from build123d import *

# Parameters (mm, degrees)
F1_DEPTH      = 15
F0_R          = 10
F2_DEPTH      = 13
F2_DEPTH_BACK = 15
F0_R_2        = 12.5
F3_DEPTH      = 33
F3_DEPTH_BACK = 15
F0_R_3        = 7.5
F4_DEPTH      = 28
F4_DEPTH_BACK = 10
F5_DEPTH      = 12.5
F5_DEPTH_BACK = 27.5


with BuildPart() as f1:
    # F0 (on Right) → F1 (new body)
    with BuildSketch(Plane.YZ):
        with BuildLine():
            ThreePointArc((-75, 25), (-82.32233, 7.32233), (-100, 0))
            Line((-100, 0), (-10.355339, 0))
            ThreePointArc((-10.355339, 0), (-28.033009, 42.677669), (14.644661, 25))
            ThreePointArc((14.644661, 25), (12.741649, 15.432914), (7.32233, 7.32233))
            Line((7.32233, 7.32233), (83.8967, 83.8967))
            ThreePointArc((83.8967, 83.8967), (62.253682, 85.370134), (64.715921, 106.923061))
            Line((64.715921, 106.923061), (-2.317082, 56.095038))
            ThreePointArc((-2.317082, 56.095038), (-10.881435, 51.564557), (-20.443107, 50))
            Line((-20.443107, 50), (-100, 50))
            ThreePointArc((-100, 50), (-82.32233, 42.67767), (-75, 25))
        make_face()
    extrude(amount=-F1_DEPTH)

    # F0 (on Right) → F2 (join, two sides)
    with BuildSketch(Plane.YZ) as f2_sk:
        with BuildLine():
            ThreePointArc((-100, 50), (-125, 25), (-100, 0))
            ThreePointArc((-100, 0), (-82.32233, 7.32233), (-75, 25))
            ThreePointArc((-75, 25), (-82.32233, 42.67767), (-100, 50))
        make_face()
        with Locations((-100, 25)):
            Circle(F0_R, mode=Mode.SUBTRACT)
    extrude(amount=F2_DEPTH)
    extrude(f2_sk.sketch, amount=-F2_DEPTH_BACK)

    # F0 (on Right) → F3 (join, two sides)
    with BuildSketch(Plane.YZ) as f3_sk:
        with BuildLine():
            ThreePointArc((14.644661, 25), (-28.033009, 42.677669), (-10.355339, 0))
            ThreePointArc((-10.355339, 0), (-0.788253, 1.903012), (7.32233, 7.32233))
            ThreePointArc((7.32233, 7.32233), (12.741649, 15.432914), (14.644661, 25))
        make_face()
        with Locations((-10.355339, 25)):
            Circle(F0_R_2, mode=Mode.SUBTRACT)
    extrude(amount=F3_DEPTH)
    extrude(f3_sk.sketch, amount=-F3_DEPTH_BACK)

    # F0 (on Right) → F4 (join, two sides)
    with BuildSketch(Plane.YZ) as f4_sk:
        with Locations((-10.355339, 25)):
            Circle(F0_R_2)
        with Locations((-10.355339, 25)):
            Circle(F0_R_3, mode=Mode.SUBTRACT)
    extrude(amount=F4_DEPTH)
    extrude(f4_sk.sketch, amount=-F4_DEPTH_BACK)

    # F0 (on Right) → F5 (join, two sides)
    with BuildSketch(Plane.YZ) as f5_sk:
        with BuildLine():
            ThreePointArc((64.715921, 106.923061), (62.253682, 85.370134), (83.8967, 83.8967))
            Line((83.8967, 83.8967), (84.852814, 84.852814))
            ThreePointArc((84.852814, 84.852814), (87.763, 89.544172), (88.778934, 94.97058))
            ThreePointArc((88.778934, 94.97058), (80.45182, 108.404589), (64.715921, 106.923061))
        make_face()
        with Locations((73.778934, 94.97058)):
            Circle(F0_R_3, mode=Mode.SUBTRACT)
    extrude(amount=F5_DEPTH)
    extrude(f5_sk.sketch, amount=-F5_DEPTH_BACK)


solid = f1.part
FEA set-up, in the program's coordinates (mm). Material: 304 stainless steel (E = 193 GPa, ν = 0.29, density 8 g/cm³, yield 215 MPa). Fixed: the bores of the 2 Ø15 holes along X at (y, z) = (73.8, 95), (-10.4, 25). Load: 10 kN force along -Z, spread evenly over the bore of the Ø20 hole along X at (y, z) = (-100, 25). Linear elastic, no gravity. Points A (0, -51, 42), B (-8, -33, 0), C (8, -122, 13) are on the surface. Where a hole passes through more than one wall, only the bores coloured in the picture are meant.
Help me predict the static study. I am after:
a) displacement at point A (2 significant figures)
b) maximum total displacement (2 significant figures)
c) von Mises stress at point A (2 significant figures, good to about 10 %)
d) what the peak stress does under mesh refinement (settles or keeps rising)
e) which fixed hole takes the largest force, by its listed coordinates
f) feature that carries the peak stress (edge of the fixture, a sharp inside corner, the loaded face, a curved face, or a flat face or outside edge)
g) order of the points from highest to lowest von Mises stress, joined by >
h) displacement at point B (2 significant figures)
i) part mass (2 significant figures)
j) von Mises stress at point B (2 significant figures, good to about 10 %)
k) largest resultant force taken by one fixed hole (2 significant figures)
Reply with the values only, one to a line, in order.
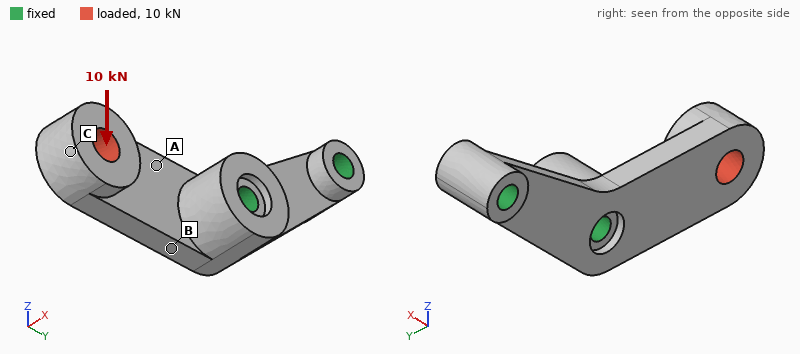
0.044 mm
0.18 mm
72 MPa
keeps rising
(-10.4, 25)
edge of the fixture
B > A > C
0.028 mm
1.8 kg
110 MPa
11 kN
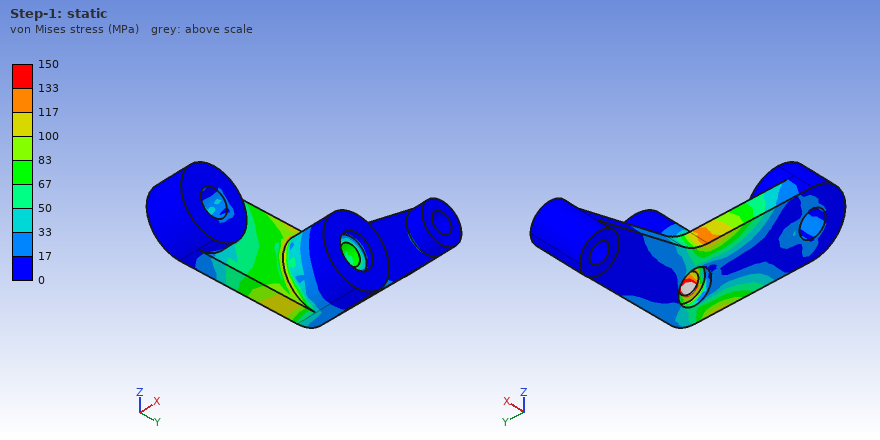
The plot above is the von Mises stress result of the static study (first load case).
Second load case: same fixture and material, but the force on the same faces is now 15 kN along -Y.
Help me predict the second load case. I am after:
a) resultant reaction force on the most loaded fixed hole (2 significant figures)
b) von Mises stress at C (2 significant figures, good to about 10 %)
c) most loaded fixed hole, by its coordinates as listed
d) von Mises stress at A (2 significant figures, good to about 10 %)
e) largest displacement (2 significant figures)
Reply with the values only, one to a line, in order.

15 kN
7.7 MPa
(-10.4, 25)
70 MPa
0.14 mm
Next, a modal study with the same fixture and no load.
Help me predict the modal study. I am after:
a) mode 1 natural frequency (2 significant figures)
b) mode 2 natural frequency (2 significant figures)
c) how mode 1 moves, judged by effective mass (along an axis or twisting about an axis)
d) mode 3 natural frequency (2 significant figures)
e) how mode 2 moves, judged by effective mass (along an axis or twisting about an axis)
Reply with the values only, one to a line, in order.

1000 Hz
2100 Hz
along X
3700 Hz
along Z
